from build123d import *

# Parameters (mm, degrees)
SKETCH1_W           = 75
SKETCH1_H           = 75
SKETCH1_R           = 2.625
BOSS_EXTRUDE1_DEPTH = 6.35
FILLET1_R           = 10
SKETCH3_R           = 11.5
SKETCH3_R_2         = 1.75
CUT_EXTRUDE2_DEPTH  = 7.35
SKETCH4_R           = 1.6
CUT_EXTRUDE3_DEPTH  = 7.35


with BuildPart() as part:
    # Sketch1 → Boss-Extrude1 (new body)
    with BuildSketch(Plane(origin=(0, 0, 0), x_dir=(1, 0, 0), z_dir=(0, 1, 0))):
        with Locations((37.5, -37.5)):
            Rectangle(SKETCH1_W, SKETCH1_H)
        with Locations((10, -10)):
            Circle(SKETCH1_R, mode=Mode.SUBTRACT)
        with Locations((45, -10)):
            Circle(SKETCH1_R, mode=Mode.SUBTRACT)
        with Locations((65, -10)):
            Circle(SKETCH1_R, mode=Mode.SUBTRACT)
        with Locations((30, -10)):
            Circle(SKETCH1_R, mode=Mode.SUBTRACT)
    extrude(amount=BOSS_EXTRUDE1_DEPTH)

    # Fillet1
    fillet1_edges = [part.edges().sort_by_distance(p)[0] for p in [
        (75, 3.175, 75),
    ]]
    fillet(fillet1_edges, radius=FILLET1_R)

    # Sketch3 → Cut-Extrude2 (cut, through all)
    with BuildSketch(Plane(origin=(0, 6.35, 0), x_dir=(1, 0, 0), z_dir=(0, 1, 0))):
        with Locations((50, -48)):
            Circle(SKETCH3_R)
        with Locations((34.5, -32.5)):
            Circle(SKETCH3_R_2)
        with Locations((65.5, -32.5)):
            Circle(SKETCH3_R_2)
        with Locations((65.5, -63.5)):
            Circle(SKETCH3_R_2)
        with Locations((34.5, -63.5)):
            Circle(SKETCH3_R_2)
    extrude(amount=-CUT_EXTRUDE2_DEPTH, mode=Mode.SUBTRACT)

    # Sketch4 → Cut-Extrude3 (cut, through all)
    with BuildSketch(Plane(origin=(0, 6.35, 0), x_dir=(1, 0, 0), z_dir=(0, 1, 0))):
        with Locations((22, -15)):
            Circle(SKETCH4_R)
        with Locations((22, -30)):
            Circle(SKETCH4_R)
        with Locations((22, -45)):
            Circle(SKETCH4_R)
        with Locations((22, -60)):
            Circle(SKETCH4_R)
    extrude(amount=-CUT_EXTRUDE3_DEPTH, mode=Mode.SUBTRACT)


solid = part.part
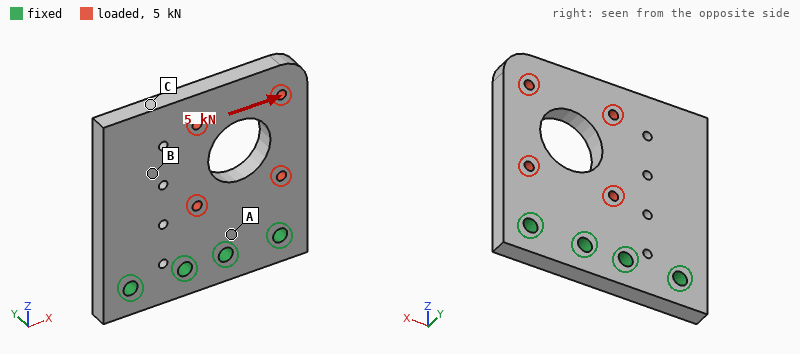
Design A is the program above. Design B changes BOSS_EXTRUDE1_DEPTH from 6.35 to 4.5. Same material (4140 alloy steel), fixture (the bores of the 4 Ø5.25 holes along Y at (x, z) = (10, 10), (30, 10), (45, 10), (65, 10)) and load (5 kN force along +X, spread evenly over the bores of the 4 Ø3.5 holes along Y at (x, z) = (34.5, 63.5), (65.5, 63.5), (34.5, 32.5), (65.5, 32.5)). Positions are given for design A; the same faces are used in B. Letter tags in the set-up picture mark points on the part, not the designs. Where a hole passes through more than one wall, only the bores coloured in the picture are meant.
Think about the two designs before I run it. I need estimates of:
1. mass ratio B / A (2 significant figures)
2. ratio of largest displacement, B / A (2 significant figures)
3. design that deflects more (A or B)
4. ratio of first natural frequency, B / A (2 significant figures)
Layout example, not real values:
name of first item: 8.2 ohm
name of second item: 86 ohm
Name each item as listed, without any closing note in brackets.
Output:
mass ratio B / A: 0.71
ratio of largest displacement, B / A: 1.4
design that deflects more: B
ratio of first natural frequency, B / A: 0.72
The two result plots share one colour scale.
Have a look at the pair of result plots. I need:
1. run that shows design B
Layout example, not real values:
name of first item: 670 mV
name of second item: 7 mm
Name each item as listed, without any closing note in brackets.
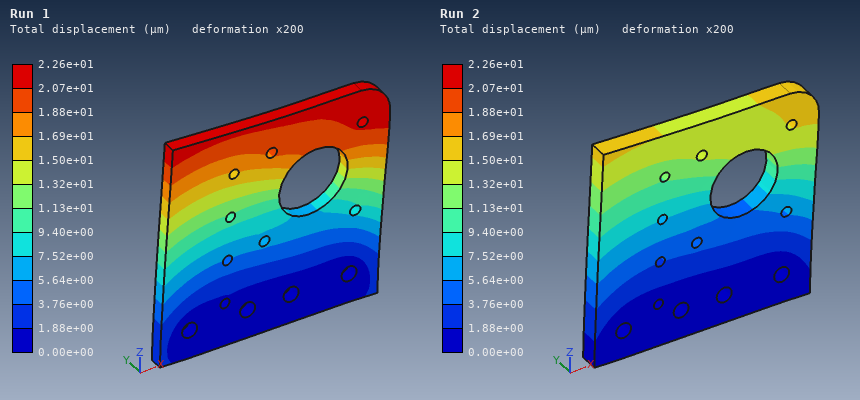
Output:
run that shows design B: Run 1
